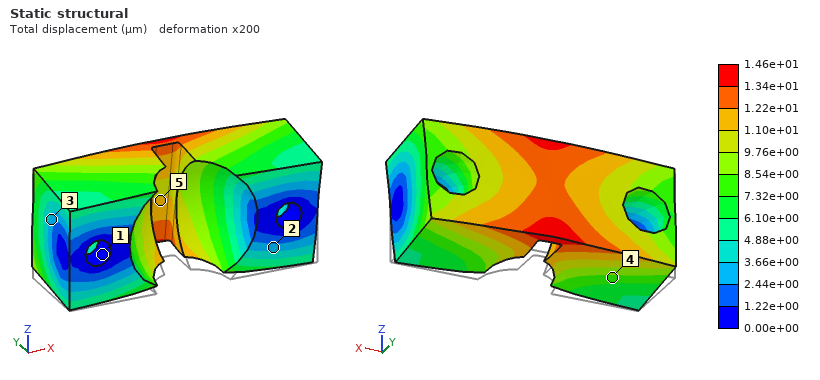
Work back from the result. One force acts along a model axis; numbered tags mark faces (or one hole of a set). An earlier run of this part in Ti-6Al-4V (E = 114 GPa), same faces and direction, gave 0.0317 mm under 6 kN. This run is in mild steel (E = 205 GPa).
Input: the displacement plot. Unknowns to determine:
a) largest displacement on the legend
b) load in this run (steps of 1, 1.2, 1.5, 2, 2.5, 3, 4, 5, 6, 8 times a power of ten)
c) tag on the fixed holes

1.46e+01 µm
5 kN
1
